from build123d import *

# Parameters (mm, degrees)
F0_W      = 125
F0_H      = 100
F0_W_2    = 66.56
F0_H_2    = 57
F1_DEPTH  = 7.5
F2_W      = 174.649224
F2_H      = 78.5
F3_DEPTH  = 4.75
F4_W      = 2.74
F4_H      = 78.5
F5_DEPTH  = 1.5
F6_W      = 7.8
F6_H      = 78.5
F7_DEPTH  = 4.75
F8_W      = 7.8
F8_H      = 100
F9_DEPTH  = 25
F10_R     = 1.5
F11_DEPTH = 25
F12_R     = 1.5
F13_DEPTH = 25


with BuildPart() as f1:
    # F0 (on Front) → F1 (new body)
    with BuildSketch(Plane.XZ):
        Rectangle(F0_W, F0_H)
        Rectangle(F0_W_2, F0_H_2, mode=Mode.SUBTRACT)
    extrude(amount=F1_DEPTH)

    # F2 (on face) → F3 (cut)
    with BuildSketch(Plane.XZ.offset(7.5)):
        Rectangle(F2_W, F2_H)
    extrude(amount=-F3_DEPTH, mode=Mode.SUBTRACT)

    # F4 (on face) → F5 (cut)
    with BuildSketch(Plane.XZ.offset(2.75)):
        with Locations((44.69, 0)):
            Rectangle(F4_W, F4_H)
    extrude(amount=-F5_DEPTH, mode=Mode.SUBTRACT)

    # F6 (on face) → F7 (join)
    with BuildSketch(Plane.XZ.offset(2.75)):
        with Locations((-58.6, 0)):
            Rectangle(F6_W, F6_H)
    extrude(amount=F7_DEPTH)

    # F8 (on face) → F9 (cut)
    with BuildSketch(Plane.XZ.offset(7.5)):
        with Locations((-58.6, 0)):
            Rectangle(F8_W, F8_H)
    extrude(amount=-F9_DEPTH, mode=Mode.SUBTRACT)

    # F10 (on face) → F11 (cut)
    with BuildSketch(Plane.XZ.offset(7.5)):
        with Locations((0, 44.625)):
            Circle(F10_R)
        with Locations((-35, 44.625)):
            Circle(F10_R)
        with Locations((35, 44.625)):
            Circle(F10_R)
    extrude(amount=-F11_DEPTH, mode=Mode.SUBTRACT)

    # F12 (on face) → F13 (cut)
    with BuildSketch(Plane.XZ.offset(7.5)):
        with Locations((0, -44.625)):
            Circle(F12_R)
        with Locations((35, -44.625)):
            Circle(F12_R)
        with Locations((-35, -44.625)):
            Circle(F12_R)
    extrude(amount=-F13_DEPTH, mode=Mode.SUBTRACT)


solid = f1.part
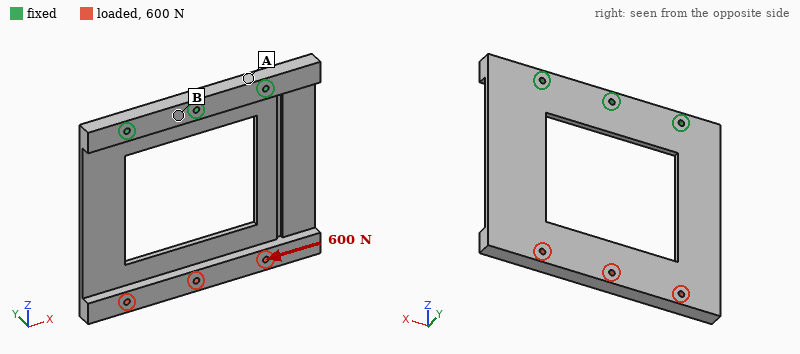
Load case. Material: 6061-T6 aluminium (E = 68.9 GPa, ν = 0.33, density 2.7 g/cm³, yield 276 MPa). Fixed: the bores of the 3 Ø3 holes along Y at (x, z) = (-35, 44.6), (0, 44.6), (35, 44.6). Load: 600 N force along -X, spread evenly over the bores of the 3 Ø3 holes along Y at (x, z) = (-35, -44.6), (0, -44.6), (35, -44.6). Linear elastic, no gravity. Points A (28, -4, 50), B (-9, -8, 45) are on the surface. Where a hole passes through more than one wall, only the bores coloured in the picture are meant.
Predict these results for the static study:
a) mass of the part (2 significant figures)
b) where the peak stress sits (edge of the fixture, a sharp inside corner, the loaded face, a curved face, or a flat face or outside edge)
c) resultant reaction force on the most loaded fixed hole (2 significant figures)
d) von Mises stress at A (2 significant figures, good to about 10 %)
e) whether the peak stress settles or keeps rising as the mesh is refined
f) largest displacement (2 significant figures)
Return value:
89 g
edge of the fixture
780 N
16 MPa
keeps rising
0.34 mm
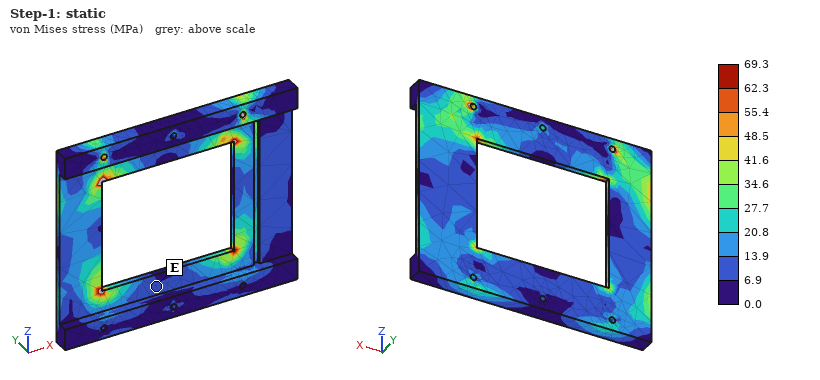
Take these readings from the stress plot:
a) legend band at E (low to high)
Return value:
6.9 to 13.9 MPa
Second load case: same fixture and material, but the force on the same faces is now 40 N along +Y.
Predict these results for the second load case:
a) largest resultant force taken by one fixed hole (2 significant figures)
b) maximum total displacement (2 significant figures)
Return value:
28 N
1.5 mm
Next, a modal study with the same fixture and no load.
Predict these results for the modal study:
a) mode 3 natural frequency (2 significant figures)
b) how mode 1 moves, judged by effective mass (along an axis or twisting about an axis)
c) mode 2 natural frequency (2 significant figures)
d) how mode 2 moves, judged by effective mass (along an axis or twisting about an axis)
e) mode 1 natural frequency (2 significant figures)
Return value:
1400 Hz
along Y
410 Hz
twisting about Z
150 Hz
